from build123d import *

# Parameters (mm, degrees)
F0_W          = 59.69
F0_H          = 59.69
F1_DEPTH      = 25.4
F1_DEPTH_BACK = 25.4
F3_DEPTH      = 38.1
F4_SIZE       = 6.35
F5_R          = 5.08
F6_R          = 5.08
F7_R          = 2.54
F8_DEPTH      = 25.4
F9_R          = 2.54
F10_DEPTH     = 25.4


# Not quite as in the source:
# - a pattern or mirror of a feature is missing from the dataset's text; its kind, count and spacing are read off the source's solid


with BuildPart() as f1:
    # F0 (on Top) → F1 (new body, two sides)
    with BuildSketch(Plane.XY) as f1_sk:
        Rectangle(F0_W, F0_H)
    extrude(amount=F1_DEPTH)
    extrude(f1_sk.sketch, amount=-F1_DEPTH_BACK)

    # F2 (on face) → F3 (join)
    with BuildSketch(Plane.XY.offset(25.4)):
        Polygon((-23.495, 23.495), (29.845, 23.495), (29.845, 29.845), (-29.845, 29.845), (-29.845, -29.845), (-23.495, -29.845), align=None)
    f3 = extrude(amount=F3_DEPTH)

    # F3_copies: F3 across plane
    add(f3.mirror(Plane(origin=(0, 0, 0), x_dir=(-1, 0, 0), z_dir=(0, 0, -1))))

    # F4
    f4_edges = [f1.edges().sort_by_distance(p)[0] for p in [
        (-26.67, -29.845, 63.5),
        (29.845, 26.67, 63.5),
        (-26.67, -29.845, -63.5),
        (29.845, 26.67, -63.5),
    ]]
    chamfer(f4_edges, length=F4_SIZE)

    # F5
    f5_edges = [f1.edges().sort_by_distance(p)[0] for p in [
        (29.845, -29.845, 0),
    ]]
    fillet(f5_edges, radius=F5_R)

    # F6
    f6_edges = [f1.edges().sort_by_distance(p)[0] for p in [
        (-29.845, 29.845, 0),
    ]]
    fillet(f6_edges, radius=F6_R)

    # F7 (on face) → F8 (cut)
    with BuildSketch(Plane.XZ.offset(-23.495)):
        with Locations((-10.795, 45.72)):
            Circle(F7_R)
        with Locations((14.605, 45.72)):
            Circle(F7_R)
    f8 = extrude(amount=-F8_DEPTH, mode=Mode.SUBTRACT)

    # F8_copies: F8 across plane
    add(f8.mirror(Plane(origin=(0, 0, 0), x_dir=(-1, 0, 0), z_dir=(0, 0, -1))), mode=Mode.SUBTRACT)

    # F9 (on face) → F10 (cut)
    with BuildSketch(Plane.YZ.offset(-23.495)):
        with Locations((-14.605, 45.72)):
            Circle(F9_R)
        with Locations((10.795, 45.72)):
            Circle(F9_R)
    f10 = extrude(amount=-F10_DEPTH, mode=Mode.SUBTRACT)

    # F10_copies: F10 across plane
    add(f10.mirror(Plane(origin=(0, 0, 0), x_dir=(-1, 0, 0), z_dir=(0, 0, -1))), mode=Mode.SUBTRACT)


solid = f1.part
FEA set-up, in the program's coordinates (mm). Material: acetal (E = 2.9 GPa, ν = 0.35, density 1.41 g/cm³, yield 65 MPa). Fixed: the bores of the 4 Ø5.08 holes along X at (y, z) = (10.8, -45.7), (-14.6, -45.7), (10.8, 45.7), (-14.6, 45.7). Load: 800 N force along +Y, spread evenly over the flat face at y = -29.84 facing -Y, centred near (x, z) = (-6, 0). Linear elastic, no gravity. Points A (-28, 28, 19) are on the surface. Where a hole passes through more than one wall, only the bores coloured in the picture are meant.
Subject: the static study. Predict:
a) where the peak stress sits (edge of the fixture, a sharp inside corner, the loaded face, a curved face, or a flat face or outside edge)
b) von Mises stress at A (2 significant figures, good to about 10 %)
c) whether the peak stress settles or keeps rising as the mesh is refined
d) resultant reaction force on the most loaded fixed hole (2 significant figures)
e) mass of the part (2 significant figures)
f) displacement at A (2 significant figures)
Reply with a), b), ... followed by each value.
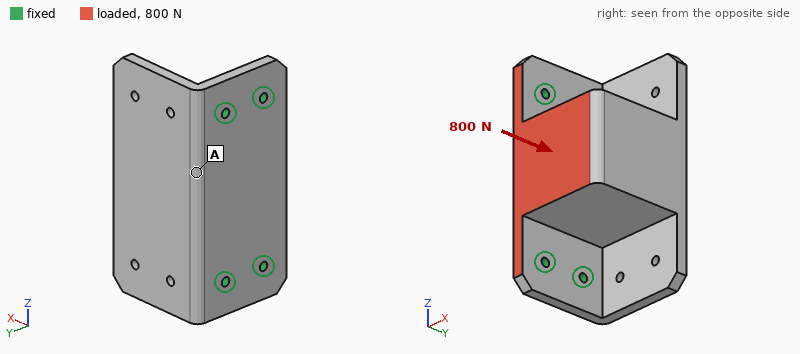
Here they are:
a) edge of the fixture
b) 2.1 MPa
c) keeps rising
d) 380 N
e) 330 g
f) 0.17 mm
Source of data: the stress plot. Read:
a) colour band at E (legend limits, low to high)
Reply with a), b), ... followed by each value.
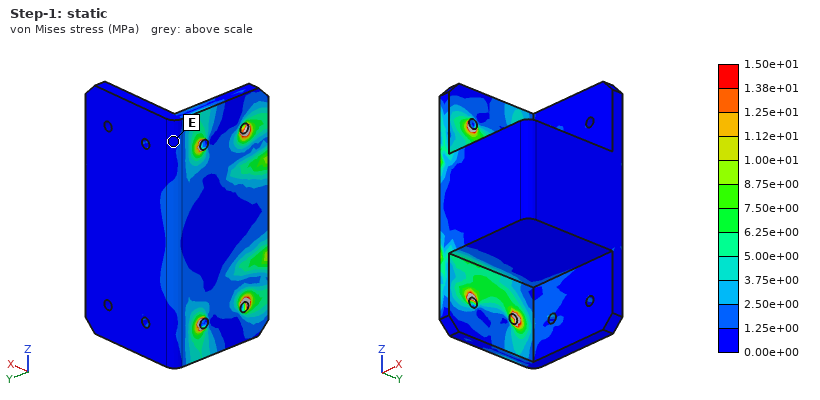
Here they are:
a) 0.00e+00 to 1.25e+00 MPa
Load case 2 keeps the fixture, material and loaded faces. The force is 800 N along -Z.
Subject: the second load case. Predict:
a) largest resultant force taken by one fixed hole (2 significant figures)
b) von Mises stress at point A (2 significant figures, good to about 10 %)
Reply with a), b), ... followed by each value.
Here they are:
a) 280 N
b) 1.2 MPa
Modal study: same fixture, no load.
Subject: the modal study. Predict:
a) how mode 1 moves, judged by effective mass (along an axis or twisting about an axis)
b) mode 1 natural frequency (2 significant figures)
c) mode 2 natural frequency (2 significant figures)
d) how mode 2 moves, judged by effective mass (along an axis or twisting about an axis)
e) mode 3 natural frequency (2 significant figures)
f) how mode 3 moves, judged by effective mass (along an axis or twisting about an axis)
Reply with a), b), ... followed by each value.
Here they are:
a) along Y
b) 370 Hz
c) 810 Hz
d) along X
e) 860 Hz
f) along Z
